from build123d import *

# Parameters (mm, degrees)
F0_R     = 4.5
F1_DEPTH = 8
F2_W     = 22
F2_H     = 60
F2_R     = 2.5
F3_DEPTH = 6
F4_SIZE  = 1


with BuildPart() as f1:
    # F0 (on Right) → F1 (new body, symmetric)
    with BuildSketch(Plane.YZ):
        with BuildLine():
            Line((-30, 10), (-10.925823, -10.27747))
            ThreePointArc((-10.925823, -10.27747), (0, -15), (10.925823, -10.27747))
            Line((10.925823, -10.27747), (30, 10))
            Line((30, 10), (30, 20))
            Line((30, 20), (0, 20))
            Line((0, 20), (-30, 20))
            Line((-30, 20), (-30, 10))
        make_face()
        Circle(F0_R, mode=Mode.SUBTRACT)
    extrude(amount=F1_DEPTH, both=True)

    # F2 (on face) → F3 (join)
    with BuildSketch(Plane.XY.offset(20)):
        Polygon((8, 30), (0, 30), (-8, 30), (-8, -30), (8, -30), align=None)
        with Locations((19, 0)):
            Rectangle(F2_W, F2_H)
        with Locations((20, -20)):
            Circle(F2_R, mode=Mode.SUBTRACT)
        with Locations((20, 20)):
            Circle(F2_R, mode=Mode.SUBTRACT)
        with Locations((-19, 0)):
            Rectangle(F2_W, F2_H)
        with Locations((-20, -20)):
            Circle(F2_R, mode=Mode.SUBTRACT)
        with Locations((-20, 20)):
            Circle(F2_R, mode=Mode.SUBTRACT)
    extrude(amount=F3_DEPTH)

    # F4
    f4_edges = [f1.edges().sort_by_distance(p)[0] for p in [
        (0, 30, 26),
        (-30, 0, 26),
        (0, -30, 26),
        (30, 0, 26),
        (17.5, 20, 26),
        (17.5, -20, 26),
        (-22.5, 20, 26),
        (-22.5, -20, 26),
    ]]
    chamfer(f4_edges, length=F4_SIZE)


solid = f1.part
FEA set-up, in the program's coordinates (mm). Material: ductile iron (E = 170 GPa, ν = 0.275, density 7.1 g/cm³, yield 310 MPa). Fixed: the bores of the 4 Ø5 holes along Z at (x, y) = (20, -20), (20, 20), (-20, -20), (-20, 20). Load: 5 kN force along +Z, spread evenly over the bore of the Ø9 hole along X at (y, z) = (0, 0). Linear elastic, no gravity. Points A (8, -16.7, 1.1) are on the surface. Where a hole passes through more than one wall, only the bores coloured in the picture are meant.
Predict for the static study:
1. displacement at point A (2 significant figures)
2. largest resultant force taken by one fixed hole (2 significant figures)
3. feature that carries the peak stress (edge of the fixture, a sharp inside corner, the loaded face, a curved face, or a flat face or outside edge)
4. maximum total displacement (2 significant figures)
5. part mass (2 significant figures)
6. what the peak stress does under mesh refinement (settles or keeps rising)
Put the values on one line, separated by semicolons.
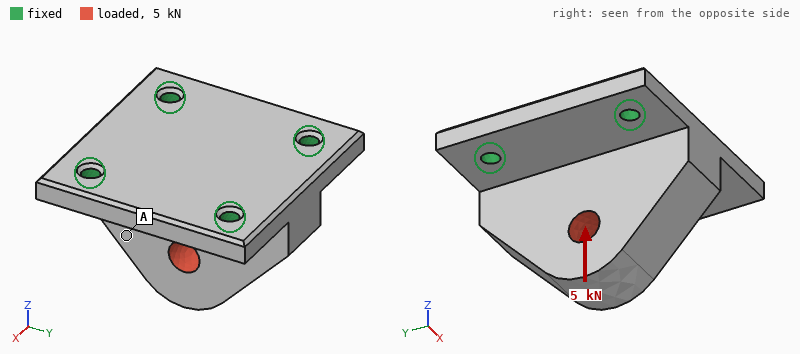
8.2 µm; 1.3 kN; edge of the fixture; 9.7 µm; 310 g; keeps rising
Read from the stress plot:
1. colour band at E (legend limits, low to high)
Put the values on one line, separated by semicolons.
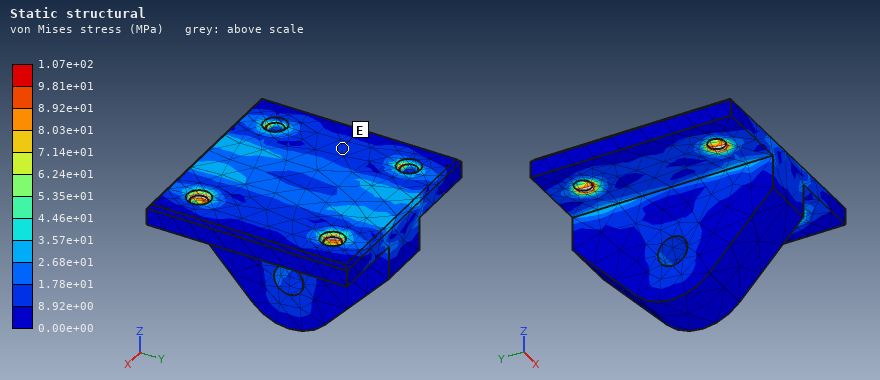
8.92e+00 to 1.78e+01 MPa
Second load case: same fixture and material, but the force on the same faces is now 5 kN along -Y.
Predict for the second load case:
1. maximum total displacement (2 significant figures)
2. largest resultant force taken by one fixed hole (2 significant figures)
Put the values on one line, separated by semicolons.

21 µm; 1.9 kN
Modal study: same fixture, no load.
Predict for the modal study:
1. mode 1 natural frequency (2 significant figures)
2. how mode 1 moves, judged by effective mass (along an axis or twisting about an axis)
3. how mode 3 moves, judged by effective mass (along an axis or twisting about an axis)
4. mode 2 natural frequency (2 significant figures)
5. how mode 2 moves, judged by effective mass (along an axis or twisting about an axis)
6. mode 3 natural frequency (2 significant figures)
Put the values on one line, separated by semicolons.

6500 Hz; along X; along Z; 7300 Hz; along Y; 8400 Hz
